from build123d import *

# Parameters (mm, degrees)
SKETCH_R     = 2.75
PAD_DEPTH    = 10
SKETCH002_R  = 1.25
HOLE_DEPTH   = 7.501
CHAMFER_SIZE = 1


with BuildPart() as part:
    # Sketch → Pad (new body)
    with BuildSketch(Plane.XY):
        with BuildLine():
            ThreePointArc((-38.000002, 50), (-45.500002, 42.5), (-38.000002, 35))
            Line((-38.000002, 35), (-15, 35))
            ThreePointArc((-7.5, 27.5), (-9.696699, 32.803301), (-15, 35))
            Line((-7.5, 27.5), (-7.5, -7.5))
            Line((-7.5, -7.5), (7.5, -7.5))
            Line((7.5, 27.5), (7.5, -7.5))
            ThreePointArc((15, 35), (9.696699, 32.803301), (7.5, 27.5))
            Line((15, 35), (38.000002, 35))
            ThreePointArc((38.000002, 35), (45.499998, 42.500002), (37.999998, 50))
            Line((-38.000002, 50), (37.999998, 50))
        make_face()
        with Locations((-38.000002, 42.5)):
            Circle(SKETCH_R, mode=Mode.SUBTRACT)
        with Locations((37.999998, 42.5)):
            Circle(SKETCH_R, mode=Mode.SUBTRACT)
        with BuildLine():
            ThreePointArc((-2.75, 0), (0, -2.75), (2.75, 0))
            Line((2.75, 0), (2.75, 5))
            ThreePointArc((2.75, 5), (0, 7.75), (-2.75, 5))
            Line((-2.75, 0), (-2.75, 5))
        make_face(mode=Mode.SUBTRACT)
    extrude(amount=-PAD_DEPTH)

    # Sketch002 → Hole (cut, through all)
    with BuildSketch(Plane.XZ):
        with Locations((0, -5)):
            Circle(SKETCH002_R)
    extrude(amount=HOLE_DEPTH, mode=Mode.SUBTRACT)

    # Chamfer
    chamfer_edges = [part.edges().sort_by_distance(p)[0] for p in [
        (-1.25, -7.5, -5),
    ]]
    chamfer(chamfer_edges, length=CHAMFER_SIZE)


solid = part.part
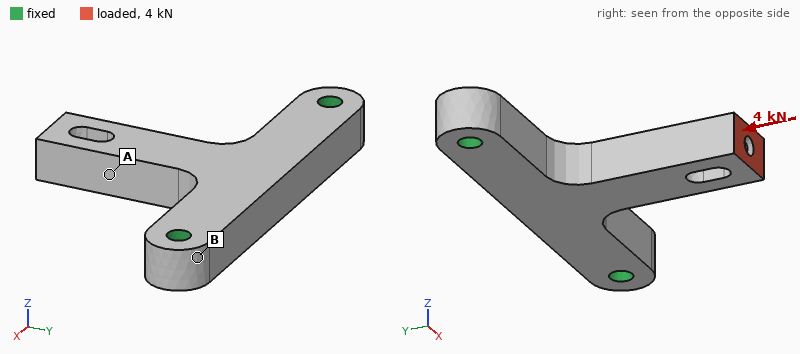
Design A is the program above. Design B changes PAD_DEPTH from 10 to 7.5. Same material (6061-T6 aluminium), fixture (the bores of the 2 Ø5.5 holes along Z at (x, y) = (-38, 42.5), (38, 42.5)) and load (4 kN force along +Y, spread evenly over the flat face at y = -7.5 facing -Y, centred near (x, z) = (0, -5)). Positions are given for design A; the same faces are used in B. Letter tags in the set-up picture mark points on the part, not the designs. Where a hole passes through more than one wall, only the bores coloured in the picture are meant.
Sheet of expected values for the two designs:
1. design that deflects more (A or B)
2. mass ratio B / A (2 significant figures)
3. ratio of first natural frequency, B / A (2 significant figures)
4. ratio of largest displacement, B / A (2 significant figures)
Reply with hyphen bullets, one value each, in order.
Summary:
- B
- 0.75
- 0.80
- 1.5
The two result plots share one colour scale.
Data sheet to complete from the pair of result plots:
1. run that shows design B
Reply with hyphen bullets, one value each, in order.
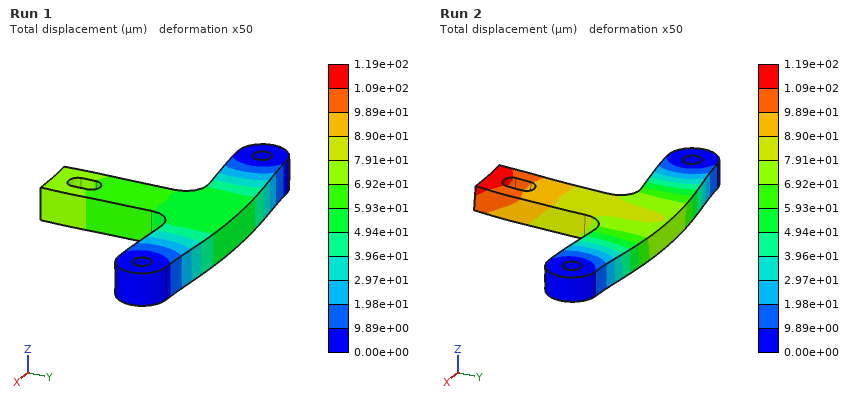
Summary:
- Run 2
